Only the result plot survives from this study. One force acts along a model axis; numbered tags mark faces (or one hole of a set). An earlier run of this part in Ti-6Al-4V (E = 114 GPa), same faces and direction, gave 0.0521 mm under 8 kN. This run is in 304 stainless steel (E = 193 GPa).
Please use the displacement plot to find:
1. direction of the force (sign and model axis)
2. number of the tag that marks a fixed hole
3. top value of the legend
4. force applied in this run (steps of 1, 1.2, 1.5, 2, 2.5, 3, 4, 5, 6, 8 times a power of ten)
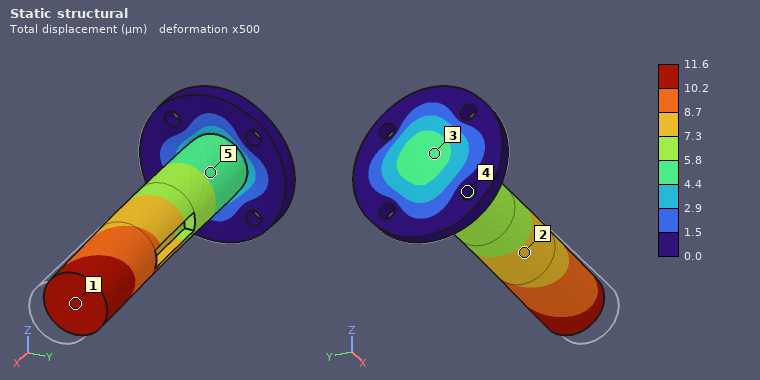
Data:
-X
4
11.6 µm
3 kN
